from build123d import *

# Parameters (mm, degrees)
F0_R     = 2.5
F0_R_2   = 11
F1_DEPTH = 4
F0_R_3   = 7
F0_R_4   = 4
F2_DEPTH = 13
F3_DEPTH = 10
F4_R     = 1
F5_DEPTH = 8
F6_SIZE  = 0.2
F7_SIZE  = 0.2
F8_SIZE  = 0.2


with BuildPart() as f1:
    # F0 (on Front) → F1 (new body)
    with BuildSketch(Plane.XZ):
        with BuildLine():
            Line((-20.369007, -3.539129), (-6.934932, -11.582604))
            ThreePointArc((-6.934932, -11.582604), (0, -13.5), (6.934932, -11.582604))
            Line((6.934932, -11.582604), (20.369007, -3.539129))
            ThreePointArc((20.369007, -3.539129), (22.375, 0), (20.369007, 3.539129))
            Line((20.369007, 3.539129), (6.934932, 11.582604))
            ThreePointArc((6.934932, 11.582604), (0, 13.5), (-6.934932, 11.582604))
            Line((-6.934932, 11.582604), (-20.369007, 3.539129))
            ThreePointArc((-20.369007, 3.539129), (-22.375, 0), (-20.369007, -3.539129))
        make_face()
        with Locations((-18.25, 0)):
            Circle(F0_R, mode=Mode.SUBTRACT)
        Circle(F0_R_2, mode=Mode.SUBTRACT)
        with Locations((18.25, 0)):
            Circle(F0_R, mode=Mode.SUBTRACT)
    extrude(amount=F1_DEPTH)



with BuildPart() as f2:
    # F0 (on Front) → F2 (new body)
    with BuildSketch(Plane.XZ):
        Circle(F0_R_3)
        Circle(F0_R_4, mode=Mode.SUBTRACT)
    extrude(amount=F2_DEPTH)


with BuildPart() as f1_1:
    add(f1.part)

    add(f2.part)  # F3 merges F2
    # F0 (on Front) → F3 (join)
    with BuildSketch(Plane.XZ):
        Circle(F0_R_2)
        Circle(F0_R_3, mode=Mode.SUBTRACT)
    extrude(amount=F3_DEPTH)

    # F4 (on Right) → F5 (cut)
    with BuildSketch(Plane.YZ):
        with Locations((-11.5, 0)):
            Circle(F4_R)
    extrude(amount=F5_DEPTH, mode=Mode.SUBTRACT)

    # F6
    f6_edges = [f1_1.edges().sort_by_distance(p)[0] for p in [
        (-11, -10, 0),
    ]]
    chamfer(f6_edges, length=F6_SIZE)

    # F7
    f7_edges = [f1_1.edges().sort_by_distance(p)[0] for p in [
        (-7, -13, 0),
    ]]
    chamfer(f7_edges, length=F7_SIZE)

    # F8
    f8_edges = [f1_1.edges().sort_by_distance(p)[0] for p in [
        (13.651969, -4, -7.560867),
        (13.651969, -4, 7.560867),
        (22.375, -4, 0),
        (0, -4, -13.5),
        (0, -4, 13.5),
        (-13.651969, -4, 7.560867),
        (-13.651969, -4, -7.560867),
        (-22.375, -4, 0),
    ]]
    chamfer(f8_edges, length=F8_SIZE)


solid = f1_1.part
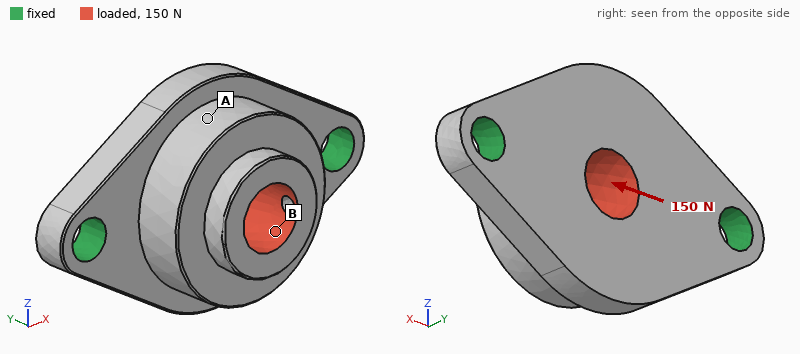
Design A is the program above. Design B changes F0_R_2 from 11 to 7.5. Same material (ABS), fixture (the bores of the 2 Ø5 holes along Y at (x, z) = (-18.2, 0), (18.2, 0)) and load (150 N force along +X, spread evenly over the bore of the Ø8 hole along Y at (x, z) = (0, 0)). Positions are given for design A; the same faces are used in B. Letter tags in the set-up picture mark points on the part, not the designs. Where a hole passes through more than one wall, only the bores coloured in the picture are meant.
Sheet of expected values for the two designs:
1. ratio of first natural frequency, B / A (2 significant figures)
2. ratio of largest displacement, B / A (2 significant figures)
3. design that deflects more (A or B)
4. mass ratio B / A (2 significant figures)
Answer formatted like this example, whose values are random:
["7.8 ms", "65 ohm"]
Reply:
["1.1", "2.3", "B", "0.76"]
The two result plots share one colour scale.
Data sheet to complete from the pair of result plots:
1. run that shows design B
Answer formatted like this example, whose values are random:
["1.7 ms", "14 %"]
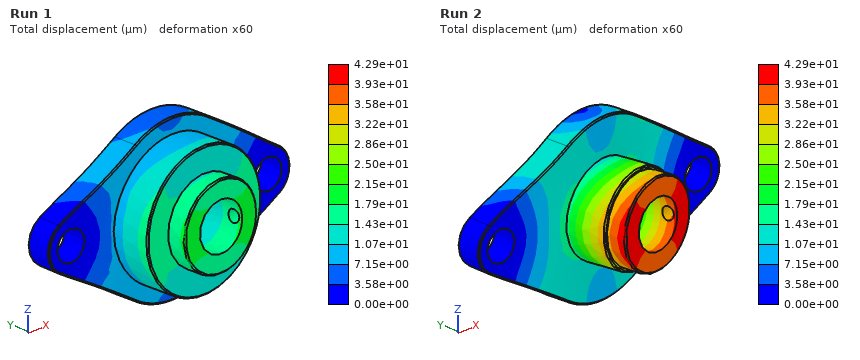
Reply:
["Run 2"]
